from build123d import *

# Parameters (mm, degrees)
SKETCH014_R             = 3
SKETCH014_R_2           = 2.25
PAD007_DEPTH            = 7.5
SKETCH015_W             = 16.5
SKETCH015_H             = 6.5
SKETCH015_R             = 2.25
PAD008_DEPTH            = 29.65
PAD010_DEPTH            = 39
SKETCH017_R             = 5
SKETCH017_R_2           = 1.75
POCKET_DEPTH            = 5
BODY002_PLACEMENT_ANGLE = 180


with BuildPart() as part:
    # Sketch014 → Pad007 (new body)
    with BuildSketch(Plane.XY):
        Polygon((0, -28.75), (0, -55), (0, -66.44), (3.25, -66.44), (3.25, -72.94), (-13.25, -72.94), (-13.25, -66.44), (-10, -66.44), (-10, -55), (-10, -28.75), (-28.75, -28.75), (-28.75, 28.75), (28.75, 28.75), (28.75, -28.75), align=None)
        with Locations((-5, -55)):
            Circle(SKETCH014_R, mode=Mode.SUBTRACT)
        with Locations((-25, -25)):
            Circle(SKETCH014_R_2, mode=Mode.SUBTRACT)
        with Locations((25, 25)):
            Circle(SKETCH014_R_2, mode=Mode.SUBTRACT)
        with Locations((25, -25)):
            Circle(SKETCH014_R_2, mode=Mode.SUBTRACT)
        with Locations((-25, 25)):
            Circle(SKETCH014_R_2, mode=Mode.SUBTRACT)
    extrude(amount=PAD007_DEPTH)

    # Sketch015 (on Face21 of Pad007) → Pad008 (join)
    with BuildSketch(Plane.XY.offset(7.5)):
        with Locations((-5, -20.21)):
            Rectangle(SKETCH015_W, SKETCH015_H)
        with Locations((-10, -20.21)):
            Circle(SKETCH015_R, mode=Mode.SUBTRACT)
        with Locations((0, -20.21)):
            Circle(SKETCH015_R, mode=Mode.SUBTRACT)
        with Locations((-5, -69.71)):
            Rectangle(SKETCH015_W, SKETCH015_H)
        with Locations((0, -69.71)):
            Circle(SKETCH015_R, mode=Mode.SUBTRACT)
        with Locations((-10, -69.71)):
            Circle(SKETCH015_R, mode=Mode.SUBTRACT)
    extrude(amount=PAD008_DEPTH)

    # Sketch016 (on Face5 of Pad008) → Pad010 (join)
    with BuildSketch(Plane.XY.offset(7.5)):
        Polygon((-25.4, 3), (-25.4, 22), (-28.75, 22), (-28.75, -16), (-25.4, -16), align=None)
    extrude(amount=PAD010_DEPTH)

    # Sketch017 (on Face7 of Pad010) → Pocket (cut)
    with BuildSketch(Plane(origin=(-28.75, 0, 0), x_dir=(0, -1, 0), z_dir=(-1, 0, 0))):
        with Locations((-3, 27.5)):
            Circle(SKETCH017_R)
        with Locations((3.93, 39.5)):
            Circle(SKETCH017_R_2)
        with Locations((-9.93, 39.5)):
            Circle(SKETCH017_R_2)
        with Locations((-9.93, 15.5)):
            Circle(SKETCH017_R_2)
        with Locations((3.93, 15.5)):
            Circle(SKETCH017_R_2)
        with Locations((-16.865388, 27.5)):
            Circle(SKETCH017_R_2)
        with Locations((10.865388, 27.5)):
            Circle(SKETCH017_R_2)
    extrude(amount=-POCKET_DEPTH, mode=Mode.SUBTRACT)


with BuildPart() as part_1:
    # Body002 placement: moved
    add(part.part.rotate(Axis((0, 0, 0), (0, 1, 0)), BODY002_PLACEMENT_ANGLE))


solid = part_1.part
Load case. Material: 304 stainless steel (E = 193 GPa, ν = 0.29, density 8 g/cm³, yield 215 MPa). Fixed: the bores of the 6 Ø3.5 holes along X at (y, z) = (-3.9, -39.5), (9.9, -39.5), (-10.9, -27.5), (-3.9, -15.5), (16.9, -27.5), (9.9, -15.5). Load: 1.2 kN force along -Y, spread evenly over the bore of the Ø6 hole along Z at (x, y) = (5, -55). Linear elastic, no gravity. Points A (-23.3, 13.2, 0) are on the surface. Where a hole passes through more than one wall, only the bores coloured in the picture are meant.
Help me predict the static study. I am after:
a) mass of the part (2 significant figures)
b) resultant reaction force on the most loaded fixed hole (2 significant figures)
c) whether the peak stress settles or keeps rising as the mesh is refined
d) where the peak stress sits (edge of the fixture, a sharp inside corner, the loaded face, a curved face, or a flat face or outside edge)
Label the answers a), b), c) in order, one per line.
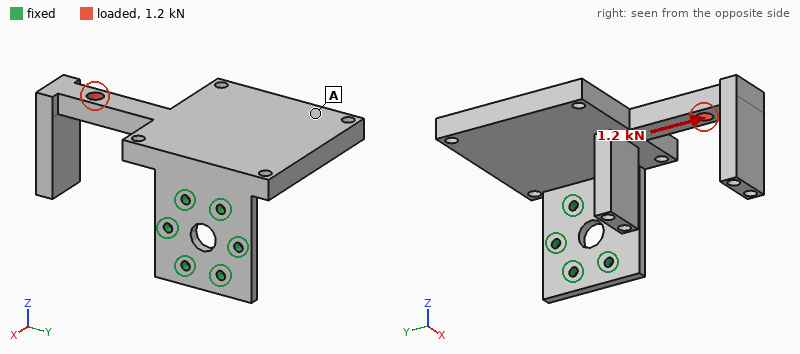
a) 290 g
b) 1.5 kN
c) keeps rising
d) edge of the fixture
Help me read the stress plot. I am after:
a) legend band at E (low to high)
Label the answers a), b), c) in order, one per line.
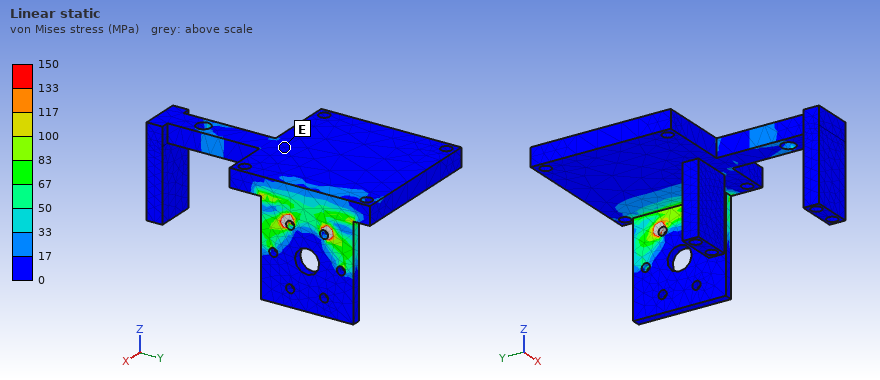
a) 0 to 17 MPa
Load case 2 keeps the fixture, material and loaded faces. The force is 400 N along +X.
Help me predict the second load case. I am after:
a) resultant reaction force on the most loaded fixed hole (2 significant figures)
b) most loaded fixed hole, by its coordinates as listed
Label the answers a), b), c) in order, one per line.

a) 1.4 kN
b) (-3.9, -15.5)
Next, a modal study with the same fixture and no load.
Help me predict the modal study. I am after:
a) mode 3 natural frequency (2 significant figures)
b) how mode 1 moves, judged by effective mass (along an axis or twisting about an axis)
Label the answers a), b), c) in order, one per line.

a) 970 Hz
b) along Z
